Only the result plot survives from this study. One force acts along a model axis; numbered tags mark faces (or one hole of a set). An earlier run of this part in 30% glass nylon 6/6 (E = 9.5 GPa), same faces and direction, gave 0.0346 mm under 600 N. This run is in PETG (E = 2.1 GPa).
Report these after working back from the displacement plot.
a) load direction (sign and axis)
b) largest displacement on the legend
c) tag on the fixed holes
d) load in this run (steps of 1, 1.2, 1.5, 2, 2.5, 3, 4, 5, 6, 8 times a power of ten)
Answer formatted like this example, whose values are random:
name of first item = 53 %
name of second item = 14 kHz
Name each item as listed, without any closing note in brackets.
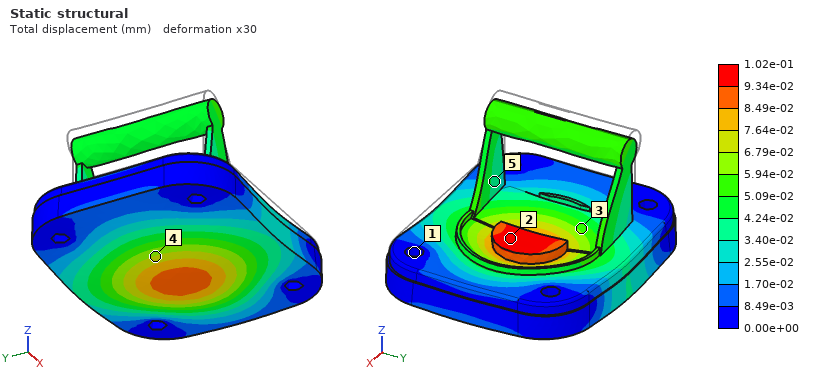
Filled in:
load direction = -Z
largest displacement on the legend = 1.02e-01 mm
tag on the fixed holes = 1
load in this run = 400 N
